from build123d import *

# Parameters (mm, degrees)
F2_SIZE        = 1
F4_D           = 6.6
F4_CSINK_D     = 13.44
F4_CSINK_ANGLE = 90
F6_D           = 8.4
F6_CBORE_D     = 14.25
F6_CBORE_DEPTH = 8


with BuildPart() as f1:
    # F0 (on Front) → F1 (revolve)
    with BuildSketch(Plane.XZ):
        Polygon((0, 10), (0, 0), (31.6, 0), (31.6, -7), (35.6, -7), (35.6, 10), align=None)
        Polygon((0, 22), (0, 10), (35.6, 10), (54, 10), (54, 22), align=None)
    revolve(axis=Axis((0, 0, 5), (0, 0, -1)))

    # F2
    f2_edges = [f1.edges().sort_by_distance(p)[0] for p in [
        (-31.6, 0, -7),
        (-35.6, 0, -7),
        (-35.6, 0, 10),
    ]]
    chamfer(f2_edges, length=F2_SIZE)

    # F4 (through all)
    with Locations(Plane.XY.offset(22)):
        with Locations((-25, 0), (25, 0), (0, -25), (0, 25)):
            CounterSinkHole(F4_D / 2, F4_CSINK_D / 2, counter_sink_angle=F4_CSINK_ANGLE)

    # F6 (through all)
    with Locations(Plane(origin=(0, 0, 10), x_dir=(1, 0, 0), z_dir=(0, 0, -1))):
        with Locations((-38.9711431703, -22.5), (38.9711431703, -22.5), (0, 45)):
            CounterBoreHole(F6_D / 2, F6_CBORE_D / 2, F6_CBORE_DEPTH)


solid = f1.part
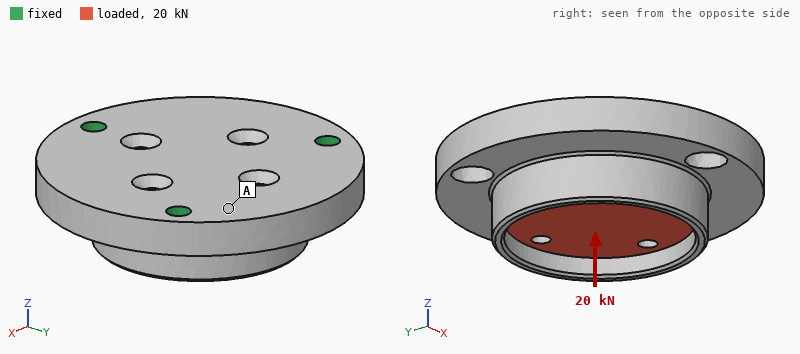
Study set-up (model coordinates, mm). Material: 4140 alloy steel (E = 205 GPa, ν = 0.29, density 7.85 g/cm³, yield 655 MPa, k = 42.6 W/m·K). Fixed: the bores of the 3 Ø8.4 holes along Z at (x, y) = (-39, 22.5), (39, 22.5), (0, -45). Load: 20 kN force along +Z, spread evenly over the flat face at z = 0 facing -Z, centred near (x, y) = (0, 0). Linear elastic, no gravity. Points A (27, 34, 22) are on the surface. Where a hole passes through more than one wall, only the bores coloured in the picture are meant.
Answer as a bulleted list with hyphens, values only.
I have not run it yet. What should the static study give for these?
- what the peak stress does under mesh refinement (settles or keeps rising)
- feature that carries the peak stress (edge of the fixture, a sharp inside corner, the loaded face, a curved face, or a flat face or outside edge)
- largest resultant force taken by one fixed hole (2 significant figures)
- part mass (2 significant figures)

- keeps rising
- edge of the fixture
- 8.2 kN
- 1.2 kg
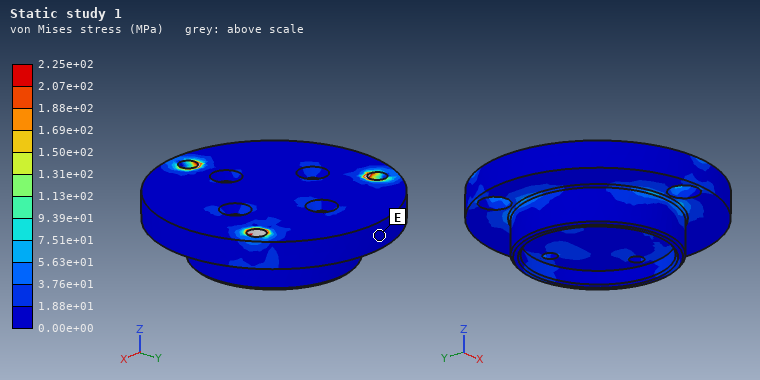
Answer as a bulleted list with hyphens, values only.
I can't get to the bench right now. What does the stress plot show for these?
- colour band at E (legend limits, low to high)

- 0.00e+00 to 1.88e+01 MPa
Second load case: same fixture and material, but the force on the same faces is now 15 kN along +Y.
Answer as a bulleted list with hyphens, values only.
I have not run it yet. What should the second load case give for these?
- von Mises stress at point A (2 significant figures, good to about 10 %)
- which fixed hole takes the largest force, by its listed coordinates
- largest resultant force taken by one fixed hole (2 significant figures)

- 13 MPa
- (0, -45)
- 8.2 kN
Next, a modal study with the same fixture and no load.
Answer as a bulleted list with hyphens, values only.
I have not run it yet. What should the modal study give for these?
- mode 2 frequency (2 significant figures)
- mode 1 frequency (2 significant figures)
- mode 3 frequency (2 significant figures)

- 6100 Hz
- 6100 Hz
- 6200 Hz
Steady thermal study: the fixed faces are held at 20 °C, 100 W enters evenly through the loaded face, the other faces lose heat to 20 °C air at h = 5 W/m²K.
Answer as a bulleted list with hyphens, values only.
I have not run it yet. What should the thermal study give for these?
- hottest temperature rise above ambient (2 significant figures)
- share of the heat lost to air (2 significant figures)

- 62 K
- 5.4 %
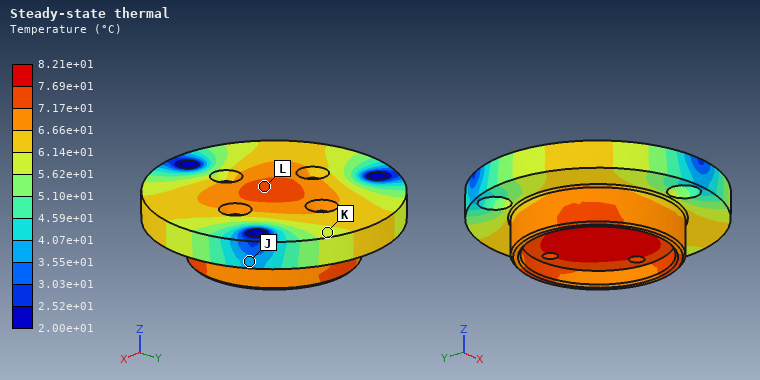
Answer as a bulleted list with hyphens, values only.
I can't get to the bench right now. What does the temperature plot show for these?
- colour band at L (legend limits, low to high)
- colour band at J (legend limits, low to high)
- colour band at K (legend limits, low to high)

- 7.17e+01 to 7.69e+01 °C
- 3.55e+01 to 4.07e+01 °C
- 5.62e+01 to 6.14e+01 °C
